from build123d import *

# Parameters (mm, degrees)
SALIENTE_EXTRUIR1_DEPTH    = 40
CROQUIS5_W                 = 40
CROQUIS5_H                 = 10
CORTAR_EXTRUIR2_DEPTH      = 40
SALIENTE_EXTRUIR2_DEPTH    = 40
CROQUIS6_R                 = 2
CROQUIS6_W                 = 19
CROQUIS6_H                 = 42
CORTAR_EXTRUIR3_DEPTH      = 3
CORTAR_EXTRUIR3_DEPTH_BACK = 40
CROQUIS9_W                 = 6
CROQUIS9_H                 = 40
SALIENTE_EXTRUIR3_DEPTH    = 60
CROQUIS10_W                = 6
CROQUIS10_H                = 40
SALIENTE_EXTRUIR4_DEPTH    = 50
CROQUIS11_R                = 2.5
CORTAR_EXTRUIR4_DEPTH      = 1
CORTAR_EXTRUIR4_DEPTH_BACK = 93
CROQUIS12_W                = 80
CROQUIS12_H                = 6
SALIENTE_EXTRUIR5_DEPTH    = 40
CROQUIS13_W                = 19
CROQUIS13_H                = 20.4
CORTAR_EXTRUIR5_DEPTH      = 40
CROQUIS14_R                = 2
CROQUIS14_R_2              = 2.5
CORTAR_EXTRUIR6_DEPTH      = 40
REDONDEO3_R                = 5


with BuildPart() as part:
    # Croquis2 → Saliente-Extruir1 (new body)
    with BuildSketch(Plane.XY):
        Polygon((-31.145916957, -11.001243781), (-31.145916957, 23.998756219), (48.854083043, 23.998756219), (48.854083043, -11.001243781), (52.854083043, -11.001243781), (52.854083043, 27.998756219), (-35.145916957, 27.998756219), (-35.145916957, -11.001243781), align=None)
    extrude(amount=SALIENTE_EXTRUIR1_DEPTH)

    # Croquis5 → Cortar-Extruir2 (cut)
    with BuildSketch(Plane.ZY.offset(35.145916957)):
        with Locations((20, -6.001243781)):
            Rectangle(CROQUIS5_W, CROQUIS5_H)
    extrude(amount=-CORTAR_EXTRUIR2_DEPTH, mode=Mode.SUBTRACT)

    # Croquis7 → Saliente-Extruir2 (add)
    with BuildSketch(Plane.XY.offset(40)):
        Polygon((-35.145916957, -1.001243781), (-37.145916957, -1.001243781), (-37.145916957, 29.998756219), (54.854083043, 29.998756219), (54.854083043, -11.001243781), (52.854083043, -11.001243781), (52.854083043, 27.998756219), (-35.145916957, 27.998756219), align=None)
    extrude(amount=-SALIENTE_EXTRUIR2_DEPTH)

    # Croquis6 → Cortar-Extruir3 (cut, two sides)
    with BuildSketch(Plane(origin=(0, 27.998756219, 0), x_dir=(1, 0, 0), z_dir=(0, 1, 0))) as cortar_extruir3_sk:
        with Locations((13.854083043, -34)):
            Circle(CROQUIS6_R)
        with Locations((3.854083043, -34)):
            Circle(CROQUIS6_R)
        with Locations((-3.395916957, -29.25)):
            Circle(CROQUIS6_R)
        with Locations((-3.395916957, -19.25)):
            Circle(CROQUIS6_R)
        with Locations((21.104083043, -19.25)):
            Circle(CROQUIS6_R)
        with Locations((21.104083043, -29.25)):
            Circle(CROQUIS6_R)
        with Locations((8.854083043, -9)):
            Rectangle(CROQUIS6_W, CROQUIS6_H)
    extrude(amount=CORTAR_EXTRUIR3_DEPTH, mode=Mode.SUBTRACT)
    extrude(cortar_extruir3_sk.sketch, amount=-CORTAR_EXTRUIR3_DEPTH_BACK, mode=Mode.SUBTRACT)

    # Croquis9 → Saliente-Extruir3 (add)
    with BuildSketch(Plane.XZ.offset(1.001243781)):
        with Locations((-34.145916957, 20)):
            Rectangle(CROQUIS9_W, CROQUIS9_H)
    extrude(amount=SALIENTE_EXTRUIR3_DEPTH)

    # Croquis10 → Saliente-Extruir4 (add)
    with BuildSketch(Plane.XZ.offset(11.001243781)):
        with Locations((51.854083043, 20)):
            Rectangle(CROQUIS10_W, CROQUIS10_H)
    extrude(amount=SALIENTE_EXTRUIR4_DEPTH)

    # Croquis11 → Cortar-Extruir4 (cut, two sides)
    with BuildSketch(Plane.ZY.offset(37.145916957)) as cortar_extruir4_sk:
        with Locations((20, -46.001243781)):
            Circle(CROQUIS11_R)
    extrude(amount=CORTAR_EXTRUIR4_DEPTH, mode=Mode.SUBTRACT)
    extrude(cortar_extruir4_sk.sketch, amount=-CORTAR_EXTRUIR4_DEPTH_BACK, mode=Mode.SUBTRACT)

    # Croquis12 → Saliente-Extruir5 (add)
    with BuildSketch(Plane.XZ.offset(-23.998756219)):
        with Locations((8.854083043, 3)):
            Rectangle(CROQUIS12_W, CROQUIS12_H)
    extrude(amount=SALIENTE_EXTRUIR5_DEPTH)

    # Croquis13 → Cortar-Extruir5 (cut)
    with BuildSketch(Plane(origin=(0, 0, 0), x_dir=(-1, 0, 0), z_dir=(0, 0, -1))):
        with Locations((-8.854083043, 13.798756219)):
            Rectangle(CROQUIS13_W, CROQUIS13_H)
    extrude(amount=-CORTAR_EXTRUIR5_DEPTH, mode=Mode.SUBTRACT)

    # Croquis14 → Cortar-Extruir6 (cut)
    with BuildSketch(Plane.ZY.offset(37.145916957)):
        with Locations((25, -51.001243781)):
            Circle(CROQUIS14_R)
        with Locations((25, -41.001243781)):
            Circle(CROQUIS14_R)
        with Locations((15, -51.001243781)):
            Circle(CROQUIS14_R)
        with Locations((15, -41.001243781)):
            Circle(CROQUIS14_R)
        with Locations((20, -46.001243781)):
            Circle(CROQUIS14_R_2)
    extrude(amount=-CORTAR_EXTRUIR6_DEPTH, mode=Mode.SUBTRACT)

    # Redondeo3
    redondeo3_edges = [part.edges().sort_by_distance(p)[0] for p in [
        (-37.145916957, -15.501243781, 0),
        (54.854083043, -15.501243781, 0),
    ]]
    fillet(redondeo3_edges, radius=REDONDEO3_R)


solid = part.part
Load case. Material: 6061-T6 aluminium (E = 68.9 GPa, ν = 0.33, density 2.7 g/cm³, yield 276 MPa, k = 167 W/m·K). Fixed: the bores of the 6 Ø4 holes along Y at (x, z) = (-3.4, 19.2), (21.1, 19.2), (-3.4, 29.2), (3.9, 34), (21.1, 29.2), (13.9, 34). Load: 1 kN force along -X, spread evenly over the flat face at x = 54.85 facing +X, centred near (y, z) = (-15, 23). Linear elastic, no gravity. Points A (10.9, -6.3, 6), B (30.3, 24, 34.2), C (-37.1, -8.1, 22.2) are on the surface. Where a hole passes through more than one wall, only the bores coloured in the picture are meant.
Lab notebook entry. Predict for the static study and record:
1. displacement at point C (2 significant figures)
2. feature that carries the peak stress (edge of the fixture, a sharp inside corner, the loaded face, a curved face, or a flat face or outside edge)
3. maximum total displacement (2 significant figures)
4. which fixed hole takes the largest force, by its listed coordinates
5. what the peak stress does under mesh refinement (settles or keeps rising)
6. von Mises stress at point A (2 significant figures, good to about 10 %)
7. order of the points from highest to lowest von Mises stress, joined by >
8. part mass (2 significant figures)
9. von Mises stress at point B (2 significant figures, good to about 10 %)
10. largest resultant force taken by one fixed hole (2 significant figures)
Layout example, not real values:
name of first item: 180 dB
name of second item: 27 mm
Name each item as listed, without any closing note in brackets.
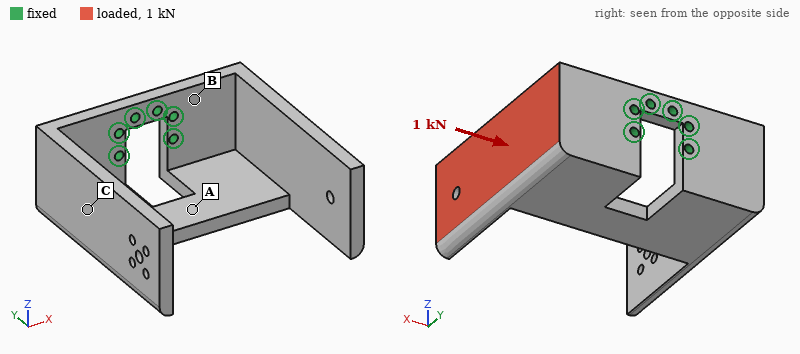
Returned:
displacement at point C: 0.15 mm
feature that carries the peak stress: edge of the fixture
maximum total displacement: 0.90 mm
which fixed hole takes the largest force, by its listed coordinates: (-3.4, 19.2)
what the peak stress does under mesh refinement: keeps rising
von Mises stress at point A: 26 MPa
order of the points from highest to lowest von Mises stress, joined by >: B > A > C
part mass: 200 g
von Mises stress at point B: 48 MPa
largest resultant force taken by one fixed hole: 1.3 kN
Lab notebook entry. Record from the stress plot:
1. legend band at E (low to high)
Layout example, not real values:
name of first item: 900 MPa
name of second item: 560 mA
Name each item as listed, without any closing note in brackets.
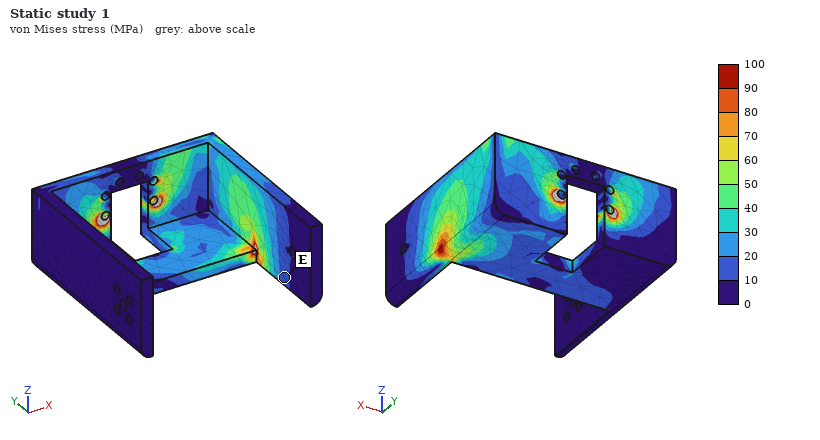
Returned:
legend band at E: 10 to 20 MPa
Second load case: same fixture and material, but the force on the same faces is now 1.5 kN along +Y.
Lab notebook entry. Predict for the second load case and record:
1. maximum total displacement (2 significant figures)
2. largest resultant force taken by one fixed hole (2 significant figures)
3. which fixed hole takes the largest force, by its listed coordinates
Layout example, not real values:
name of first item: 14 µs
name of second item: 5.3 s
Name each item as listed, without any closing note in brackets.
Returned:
maximum total displacement: 0.44 mm
largest resultant force taken by one fixed hole: 1.9 kN
which fixed hole takes the largest force, by its listed coordinates: (21.1, 19.2)
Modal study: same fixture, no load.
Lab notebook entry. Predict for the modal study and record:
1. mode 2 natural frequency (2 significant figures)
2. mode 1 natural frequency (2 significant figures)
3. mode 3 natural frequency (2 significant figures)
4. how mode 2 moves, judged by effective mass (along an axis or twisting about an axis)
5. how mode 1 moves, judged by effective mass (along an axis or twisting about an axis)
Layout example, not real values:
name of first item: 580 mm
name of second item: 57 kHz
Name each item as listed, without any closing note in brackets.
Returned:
mode 2 natural frequency: 760 Hz
mode 1 natural frequency: 690 Hz
mode 3 natural frequency: 1200 Hz
how mode 2 moves, judged by effective mass: along Z
how mode 1 moves, judged by effective mass: along X
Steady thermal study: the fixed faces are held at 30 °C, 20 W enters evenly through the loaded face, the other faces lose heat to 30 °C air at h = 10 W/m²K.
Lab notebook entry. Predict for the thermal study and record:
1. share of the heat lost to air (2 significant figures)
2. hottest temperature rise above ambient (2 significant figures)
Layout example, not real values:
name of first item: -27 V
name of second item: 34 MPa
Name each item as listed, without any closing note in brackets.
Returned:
share of the heat lost to air: 9.0 %
hottest temperature rise above ambient: 25 K
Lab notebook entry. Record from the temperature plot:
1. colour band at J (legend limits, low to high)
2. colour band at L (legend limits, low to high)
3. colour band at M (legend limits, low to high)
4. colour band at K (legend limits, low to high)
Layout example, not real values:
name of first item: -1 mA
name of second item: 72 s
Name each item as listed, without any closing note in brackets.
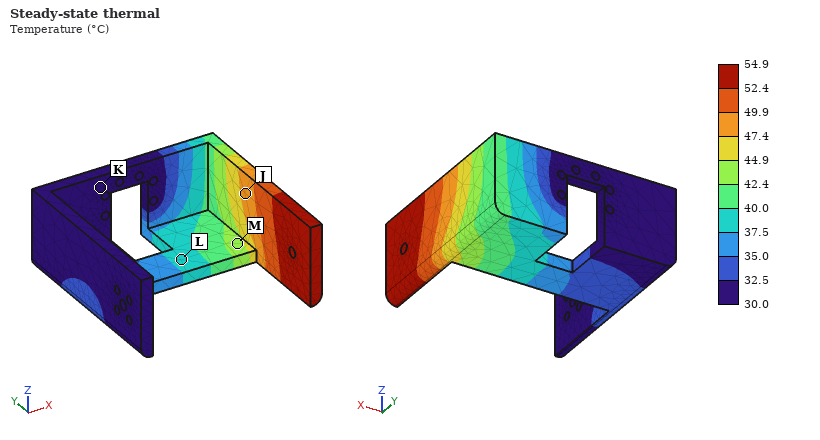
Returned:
colour band at J: 47.4 to 49.9 °C
colour band at L: 37.5 to 40.0 °C
colour band at M: 42.4 to 44.9 °C
colour band at K: 30.0 to 32.5 °C
